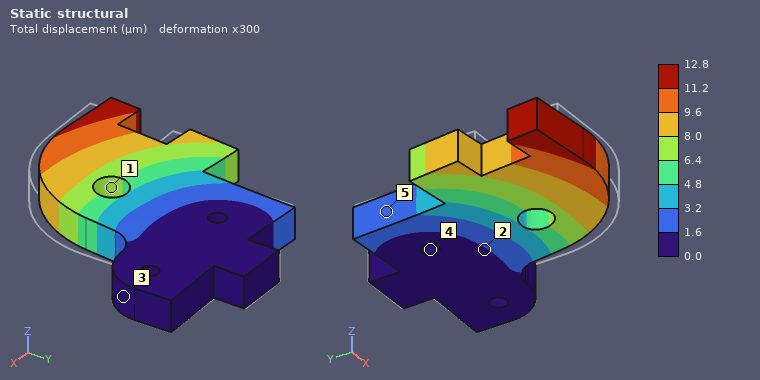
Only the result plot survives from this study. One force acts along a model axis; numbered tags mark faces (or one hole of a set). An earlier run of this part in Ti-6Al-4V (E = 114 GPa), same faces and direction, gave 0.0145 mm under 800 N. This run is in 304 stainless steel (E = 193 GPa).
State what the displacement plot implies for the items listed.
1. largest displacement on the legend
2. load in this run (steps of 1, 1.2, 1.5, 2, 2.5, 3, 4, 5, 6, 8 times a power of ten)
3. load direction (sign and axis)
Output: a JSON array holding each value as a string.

["12.8 µm", "1.2 kN", "-X"]
